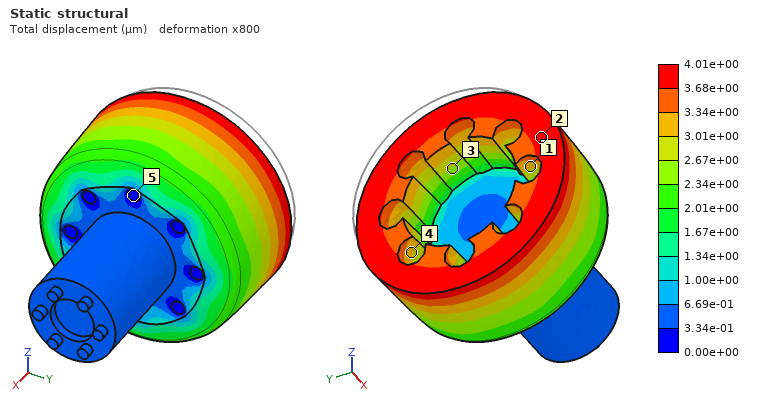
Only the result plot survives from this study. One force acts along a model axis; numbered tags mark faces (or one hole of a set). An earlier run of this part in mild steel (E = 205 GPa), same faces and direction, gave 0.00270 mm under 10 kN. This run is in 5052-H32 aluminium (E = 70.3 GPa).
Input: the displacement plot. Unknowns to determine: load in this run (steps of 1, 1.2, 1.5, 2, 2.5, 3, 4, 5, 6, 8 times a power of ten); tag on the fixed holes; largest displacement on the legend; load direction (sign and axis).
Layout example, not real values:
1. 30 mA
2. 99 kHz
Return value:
1. 5 kN
2. 5
3. 4.01e+00 µm
4. +X
